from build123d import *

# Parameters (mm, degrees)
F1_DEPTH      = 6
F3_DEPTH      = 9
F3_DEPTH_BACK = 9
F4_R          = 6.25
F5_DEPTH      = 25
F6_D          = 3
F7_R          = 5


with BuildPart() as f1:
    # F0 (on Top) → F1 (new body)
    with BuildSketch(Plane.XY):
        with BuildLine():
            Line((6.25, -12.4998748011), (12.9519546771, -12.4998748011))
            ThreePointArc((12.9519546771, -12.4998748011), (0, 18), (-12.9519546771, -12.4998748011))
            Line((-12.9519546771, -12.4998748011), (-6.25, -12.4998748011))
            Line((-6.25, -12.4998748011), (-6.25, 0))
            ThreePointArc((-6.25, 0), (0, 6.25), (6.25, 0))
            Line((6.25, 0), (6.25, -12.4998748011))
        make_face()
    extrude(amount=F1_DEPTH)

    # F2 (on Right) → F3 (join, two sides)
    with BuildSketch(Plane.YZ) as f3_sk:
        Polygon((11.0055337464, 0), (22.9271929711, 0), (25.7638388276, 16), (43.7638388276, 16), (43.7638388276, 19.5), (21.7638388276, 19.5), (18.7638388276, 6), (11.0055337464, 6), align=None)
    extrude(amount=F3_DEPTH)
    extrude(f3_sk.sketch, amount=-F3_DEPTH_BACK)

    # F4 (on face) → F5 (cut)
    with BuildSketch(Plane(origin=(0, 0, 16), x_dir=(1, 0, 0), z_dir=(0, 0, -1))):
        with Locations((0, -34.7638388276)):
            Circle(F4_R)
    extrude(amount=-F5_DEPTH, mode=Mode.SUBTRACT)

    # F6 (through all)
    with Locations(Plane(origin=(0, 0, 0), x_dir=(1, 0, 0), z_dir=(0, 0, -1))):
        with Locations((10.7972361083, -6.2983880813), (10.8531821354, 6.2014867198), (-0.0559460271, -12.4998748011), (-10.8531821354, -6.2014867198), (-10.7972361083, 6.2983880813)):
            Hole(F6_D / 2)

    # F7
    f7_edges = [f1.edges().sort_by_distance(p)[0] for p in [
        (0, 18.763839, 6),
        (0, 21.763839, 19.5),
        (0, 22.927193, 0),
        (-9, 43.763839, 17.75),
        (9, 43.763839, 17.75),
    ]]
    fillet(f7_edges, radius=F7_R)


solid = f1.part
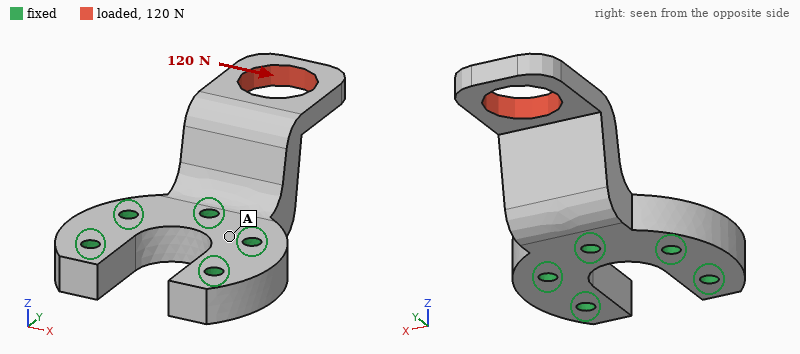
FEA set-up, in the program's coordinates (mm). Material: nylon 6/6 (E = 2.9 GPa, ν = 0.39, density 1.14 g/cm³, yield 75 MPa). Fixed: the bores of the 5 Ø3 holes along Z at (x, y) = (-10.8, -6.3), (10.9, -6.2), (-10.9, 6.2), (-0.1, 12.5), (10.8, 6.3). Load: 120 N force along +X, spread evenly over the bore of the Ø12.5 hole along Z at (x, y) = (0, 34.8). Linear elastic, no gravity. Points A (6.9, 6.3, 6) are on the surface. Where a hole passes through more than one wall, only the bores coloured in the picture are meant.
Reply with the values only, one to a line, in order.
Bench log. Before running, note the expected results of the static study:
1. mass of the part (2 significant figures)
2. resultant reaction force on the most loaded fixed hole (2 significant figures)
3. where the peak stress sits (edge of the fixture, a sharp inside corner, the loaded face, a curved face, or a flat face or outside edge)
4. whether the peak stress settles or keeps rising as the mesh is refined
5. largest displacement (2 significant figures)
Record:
7.4 g
140 N
a sharp inside corner
keeps rising
0.71 mm
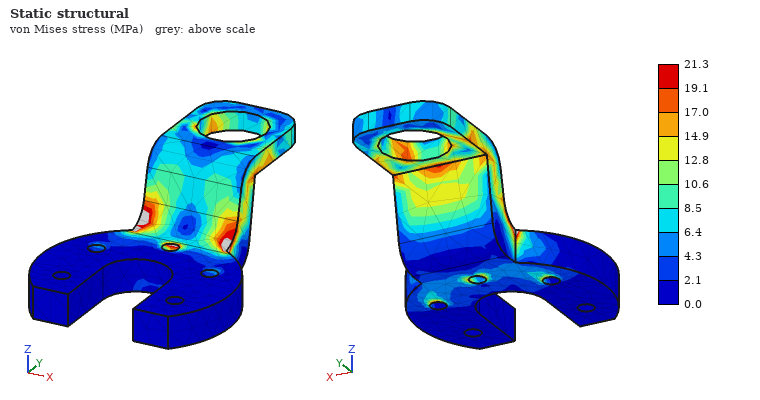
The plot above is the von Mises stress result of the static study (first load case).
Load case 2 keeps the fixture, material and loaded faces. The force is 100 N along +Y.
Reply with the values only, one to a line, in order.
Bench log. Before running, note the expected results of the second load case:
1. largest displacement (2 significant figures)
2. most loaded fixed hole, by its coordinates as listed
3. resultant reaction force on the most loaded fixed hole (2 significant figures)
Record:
0.69 mm
(-0.1, 12.5)
93 N
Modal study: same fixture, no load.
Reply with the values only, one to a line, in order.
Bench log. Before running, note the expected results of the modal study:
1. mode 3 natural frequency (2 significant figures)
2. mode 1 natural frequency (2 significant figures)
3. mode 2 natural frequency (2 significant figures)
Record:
3300 Hz
1400 Hz
2600 Hz
